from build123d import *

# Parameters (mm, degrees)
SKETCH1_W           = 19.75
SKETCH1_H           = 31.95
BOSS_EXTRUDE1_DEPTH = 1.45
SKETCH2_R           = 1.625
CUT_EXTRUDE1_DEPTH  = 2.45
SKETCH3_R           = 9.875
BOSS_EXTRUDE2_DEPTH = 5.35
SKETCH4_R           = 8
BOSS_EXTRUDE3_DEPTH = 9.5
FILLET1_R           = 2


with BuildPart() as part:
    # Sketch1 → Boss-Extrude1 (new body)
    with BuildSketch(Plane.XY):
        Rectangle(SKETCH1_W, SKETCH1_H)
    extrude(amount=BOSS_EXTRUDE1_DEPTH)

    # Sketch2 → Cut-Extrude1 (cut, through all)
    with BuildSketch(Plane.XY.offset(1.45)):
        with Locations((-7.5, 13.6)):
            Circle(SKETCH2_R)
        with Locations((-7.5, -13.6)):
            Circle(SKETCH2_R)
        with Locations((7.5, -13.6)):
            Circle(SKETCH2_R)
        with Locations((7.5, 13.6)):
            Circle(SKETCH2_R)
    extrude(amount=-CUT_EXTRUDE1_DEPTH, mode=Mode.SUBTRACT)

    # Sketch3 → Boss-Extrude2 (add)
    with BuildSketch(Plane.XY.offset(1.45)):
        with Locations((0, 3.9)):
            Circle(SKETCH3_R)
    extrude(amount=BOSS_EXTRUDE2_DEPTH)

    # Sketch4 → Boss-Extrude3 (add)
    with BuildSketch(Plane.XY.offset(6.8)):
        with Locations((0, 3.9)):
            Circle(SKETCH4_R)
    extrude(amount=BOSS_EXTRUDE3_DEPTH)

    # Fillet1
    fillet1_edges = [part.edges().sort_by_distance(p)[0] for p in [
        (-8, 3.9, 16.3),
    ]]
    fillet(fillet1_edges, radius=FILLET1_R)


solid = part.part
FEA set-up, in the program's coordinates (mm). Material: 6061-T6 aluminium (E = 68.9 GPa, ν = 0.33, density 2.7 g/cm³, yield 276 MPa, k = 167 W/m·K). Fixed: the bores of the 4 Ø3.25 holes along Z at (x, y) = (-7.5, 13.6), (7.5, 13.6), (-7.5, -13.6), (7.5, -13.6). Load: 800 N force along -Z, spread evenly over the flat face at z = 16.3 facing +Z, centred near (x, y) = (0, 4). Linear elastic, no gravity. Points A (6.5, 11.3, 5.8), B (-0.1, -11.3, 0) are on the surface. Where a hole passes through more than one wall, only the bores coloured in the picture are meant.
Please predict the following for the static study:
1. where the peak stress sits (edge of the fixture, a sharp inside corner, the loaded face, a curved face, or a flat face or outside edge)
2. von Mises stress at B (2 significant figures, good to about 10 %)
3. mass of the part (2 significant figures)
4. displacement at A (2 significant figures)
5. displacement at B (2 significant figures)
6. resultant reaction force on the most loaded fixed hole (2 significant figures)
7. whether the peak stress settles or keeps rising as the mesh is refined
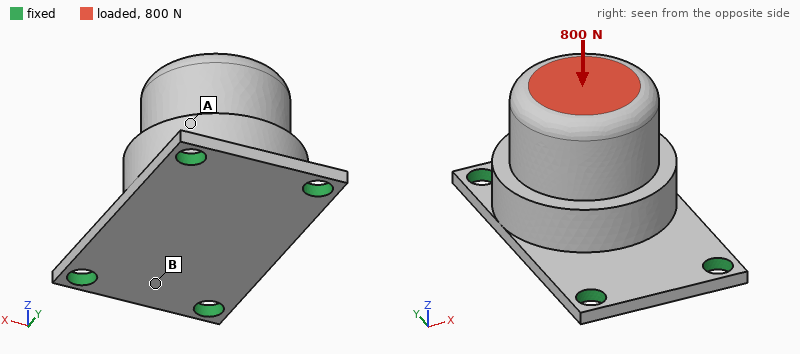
edge of the fixture
49 MPa
12 g
14 µm
18 µm
280 N
keeps rising
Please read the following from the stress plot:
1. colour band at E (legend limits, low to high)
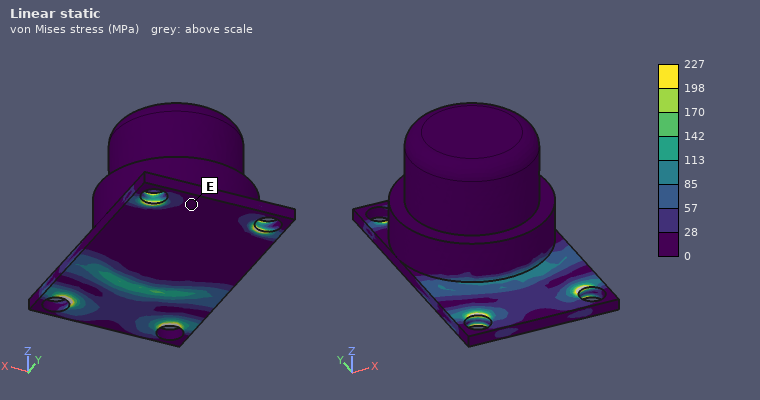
0 to 28 MPa
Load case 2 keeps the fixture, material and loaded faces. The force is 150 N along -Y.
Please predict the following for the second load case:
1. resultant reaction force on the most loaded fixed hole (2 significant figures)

69 N
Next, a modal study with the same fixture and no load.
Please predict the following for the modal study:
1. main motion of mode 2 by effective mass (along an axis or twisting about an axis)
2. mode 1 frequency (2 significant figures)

along X
6000 Hz
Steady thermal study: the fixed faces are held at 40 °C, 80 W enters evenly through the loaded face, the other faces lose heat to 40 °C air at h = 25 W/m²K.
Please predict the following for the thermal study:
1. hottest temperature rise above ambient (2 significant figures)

85 K
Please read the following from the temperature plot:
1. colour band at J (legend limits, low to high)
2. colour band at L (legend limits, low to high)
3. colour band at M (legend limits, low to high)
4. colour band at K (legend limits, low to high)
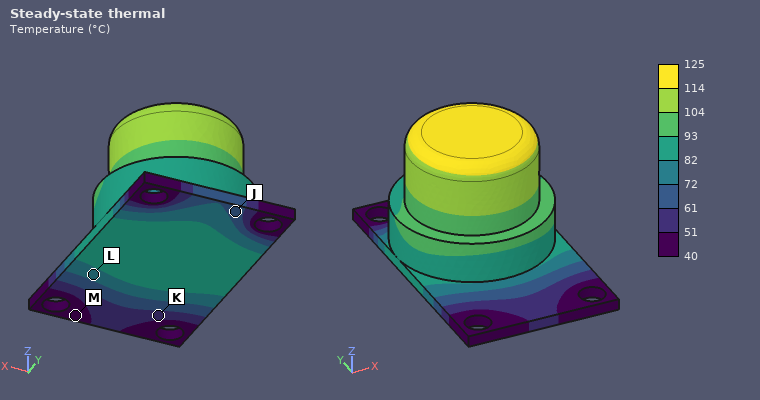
61 to 72 °C
72 to 82 °C
40 to 51 °C
51 to 61 °C
